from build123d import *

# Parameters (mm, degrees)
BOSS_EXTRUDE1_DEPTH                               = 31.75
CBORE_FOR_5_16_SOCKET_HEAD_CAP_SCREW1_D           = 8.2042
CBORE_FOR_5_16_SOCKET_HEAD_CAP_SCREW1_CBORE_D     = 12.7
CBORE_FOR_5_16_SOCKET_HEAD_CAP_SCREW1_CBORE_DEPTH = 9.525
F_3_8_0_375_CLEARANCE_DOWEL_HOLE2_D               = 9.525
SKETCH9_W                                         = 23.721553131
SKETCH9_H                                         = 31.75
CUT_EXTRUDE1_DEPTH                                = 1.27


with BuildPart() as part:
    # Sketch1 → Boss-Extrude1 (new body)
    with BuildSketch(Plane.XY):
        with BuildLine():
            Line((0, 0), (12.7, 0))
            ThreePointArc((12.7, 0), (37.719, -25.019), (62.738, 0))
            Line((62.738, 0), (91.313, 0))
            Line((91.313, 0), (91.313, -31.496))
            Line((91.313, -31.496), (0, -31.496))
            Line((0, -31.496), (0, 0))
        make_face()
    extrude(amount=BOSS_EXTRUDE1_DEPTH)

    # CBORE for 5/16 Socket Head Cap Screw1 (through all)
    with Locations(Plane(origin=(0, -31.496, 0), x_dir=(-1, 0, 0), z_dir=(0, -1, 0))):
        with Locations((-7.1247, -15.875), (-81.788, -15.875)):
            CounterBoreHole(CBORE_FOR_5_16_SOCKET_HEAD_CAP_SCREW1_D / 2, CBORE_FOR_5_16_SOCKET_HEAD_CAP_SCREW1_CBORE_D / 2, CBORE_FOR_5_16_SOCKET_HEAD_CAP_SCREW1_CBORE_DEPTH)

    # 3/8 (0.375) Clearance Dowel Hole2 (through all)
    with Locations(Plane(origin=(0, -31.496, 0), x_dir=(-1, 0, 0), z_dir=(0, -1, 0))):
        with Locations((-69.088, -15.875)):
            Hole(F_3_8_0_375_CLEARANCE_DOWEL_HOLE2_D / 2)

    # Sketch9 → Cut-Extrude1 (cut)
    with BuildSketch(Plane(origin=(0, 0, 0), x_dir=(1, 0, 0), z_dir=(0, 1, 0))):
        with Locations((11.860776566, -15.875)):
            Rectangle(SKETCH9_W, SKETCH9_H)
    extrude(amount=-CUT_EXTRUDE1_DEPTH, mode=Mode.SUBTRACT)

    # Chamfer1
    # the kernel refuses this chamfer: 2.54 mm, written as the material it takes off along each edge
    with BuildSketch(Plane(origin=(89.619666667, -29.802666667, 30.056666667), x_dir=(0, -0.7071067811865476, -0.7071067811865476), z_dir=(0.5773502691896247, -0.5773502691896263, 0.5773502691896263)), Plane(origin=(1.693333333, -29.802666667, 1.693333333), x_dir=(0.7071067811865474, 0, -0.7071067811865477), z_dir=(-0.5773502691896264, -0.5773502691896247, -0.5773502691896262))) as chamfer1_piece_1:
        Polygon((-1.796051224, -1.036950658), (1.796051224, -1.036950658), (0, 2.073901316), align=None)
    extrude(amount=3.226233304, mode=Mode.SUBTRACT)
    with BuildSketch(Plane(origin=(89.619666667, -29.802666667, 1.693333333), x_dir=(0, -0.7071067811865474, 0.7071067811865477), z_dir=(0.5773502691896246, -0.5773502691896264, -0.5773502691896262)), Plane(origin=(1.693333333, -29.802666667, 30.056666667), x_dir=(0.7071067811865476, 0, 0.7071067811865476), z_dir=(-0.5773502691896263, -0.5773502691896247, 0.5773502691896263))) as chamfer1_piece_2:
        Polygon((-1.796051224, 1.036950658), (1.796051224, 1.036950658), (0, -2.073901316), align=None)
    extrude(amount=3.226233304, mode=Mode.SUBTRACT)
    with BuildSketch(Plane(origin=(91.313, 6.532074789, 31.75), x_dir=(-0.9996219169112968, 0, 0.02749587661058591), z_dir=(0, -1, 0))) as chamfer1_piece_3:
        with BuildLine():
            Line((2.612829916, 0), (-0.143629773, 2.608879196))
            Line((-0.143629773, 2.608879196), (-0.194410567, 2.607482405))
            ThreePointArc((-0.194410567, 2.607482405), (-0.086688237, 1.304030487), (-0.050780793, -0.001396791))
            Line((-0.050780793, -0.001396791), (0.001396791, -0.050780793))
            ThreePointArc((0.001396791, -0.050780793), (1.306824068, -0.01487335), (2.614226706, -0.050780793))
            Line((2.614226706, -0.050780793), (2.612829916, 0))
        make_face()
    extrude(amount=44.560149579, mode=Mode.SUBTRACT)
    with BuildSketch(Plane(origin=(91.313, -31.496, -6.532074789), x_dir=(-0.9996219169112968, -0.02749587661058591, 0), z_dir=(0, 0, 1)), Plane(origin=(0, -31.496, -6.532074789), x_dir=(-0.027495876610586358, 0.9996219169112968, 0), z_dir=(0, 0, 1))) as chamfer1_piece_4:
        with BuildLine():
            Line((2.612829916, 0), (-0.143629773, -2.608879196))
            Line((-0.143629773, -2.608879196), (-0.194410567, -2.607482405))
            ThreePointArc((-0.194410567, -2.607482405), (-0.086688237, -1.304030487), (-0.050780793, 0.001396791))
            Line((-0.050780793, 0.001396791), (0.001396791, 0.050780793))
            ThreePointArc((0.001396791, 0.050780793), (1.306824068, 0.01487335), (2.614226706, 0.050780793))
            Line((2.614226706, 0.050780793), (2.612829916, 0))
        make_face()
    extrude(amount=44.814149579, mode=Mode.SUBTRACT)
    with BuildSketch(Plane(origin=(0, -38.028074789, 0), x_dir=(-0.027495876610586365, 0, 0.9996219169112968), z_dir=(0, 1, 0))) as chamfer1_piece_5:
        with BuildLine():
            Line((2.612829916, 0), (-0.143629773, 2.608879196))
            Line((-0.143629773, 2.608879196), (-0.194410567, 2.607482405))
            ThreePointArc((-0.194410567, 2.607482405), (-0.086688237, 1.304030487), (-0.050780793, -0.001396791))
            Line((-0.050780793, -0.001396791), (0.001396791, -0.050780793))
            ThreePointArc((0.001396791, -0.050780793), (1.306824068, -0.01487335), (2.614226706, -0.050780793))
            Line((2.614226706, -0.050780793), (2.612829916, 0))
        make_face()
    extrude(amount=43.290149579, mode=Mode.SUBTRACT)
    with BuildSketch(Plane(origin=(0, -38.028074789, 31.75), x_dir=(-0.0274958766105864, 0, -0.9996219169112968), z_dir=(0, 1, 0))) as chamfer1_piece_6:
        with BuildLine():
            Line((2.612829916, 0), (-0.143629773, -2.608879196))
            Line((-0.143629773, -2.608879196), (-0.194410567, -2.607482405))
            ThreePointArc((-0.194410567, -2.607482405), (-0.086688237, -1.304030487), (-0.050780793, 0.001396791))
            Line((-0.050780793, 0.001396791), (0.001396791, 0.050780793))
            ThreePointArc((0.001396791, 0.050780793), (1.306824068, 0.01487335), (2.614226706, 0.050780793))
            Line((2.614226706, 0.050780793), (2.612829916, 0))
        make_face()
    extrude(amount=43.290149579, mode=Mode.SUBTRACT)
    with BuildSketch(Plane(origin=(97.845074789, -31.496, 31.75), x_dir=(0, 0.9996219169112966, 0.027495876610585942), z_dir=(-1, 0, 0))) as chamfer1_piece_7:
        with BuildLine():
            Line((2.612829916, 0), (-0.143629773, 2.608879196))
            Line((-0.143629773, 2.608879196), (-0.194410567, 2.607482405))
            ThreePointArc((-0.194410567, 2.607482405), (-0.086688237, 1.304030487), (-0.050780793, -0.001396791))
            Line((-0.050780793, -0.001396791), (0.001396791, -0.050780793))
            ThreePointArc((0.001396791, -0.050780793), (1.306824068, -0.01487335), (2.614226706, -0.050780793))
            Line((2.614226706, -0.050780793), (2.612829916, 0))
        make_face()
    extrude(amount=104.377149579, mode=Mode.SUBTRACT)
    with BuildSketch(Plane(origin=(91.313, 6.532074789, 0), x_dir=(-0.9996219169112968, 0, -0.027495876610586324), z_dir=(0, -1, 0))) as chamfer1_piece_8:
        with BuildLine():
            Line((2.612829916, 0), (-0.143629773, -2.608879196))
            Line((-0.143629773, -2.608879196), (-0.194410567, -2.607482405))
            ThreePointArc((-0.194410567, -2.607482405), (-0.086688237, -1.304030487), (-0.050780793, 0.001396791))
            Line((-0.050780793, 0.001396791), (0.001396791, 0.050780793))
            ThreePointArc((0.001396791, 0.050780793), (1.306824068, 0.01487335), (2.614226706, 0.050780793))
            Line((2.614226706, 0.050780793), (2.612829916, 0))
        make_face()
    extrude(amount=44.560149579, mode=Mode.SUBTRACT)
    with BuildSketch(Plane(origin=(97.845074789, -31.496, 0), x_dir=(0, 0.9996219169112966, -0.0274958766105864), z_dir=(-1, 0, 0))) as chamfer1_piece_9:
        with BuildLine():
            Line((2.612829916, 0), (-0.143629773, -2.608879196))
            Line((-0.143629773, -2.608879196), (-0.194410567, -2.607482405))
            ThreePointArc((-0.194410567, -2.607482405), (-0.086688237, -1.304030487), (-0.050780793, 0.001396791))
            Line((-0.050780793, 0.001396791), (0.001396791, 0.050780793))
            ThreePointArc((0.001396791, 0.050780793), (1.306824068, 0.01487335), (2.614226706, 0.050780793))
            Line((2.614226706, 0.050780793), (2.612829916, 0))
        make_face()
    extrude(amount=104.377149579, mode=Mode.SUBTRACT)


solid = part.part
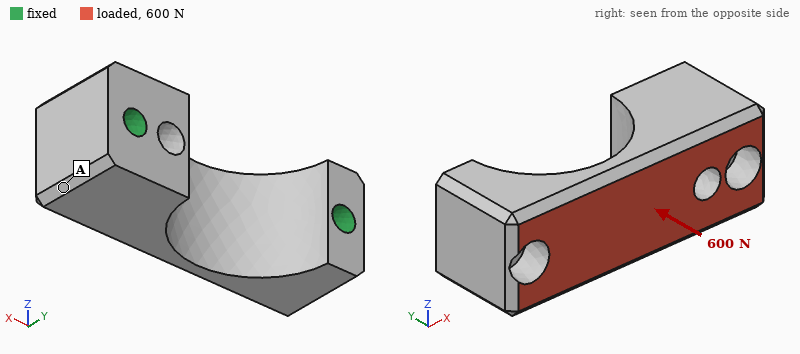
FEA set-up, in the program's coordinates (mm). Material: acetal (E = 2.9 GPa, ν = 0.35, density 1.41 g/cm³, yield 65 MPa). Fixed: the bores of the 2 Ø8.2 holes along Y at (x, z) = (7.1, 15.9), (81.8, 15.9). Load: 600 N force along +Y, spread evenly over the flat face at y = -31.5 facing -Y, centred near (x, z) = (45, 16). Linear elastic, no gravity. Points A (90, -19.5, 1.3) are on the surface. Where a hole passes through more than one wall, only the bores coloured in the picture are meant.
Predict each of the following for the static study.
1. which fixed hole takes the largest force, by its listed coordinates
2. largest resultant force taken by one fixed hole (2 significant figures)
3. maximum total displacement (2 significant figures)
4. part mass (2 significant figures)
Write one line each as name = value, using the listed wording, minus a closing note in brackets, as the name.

which fixed hole takes the largest force, by its listed coordinates = (81.8, 15.9)
largest resultant force taken by one fixed hole = 380 N
maximum total displacement = 32 µm
part mass = 73 g
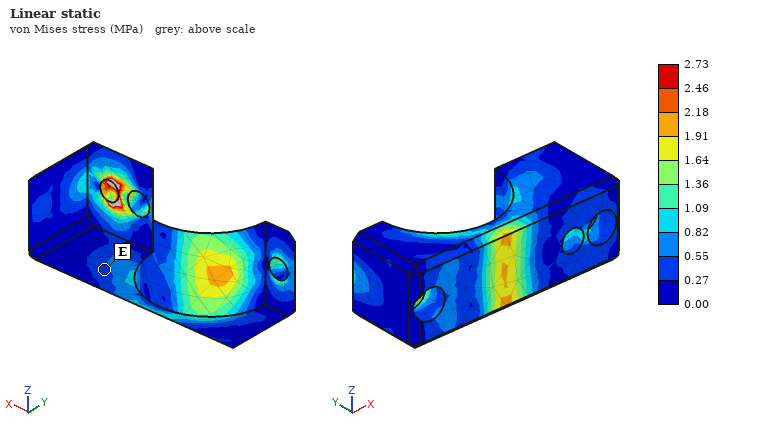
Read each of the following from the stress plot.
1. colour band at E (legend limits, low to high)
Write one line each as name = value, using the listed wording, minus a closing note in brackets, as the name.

colour band at E = 0.27 to 0.55 MPa
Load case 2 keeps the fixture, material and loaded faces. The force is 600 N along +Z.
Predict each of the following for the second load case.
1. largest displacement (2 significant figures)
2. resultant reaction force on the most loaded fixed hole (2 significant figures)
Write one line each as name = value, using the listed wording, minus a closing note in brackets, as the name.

largest displacement = 66 µm
resultant reaction force on the most loaded fixed hole = 300 N
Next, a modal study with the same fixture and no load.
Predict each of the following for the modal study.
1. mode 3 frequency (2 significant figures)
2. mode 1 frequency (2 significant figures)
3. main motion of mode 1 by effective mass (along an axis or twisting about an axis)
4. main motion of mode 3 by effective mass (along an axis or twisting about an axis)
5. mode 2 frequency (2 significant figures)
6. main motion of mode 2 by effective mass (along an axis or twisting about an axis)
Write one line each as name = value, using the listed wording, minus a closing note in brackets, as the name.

mode 3 frequency = 5400 Hz
mode 1 frequency = 3300 Hz
main motion of mode 1 by effective mass = along Z
main motion of mode 3 by effective mass = along X
mode 2 frequency = 4100 Hz
main motion of mode 2 by effective mass = along Y
